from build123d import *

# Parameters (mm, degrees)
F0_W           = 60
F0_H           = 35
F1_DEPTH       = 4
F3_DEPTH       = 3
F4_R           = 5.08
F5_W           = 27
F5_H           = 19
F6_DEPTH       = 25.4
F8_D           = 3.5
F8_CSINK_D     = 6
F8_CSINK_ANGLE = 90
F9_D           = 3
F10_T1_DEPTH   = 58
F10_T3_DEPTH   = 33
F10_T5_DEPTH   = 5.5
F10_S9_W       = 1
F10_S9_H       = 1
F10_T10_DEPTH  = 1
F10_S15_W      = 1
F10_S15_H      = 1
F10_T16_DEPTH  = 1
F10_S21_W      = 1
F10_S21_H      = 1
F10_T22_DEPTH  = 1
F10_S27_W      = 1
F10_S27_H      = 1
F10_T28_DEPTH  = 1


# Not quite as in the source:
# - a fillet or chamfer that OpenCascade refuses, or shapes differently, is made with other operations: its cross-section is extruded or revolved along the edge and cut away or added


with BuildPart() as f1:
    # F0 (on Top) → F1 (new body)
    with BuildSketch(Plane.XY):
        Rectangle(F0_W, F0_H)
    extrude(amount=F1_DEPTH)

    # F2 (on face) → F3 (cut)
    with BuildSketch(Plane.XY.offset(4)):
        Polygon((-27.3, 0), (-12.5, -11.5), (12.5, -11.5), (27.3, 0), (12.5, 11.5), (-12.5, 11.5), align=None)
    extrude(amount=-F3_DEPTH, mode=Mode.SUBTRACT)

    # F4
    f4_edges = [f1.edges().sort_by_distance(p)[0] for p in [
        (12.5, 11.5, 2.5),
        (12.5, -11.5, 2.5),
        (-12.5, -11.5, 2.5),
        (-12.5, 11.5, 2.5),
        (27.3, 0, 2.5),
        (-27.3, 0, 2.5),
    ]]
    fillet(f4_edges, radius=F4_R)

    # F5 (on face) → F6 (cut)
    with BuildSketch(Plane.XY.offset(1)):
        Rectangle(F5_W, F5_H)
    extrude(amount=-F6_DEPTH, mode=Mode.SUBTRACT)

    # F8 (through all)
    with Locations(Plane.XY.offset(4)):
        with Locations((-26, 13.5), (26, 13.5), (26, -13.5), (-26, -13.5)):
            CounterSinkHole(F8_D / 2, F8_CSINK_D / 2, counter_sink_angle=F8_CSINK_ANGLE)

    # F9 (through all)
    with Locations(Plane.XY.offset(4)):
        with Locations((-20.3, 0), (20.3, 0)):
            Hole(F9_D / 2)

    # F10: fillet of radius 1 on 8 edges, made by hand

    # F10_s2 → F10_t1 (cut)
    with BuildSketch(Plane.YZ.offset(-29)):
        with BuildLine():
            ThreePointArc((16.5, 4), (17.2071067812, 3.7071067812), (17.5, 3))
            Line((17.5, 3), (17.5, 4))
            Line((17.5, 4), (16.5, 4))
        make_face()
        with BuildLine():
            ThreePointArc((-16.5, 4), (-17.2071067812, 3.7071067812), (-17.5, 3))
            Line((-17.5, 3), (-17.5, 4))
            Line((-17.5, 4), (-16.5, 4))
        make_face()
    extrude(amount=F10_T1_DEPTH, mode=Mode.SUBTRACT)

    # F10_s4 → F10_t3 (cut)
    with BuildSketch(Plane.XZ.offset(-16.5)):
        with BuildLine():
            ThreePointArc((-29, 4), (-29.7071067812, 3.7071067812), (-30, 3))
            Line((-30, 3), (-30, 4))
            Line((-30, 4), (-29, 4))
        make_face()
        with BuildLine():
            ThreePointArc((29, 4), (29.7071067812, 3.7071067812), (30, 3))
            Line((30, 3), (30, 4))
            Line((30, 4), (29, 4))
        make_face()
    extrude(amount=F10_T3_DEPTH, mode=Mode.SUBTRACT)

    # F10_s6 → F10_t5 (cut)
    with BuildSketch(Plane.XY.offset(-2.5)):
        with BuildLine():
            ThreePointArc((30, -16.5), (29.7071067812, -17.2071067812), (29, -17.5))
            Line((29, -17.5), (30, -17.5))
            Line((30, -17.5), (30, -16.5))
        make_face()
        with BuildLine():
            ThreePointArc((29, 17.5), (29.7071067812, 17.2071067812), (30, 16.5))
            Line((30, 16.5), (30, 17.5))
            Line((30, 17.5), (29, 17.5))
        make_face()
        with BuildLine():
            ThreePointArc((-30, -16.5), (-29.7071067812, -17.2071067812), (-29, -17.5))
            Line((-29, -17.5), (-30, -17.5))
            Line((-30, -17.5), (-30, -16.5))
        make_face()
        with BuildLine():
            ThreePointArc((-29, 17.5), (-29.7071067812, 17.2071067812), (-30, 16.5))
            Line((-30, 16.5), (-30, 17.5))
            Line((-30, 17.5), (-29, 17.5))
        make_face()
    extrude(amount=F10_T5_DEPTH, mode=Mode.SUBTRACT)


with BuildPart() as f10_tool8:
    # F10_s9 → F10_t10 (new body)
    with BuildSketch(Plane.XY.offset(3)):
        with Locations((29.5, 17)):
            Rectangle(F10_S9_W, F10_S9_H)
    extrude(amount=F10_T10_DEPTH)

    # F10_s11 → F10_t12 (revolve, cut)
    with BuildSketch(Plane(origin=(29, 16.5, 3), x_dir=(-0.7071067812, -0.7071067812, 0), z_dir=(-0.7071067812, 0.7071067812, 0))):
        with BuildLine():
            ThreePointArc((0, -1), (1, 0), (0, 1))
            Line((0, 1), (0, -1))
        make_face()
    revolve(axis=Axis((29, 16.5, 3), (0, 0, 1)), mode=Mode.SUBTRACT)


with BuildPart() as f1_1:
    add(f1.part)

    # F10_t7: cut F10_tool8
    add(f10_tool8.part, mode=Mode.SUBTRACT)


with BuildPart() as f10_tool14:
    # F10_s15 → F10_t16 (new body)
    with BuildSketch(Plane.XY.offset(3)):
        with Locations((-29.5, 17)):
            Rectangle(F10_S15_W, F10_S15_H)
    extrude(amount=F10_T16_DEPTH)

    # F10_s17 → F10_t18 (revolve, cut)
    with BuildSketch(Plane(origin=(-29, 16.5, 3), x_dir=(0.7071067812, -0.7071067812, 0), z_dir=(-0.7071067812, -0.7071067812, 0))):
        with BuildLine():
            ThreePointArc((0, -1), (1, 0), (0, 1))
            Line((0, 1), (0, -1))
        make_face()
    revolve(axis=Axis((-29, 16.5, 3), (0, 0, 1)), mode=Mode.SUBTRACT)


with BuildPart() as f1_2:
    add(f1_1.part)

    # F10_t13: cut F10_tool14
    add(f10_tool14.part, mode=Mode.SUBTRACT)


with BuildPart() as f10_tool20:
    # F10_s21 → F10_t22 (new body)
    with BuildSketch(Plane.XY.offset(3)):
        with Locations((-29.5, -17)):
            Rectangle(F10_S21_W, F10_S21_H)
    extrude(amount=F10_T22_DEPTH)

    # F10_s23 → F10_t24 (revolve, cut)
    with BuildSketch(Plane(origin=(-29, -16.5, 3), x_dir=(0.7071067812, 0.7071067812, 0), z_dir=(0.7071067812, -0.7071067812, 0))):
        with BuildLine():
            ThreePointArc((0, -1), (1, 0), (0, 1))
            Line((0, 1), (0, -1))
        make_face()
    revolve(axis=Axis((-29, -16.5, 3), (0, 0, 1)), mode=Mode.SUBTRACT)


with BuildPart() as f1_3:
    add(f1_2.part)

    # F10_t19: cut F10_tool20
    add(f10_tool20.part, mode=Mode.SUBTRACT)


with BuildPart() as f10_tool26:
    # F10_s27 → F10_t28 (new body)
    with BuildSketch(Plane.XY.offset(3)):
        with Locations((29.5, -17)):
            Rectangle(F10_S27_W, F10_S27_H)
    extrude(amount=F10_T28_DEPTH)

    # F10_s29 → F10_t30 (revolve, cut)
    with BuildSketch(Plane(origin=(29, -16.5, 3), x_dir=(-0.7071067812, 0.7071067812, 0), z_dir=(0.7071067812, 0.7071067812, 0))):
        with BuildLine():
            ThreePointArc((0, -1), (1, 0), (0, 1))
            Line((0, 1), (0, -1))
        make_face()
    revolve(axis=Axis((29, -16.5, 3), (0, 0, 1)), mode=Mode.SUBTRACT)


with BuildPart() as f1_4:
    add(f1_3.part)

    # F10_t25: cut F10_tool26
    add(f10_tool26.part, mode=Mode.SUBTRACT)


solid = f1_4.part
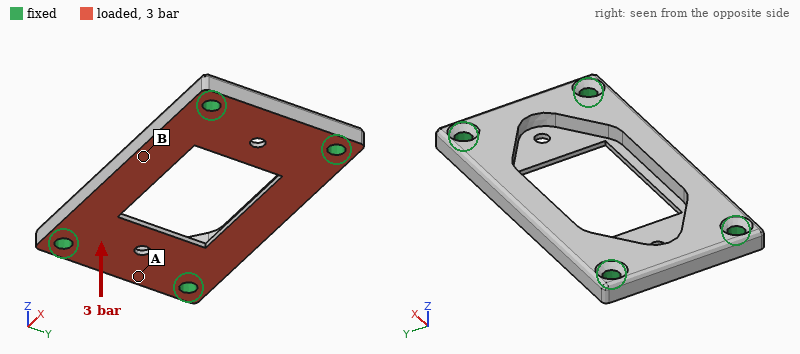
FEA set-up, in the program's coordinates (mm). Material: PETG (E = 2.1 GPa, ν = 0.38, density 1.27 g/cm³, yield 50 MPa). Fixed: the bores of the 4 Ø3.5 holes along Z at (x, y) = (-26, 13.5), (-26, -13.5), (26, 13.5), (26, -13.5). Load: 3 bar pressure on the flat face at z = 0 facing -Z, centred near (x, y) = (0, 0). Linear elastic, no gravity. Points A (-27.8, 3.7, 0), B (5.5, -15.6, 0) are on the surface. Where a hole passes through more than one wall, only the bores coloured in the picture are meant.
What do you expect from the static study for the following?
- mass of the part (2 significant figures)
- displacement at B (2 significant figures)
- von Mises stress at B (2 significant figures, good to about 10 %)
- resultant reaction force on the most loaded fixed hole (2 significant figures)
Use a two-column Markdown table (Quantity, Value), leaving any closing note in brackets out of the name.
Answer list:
| Quantity | Value |
|---|---|
| mass of the part | 6.3 g |
| displacement at B | 0.55 mm |
| von Mises stress at B | 12 MPa |
| resultant reaction force on the most loaded fixed hole | 120 N |
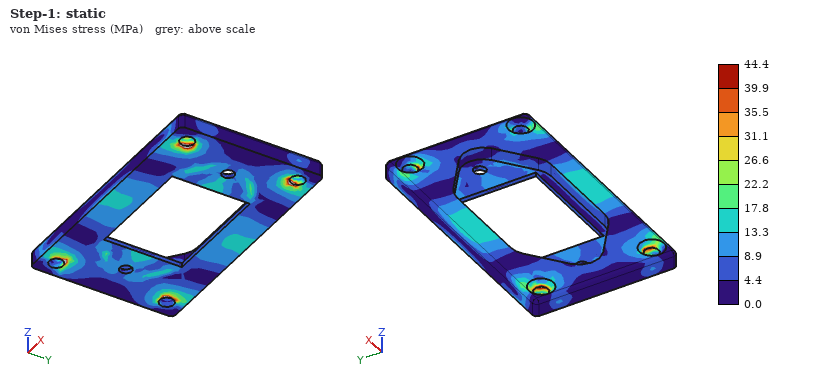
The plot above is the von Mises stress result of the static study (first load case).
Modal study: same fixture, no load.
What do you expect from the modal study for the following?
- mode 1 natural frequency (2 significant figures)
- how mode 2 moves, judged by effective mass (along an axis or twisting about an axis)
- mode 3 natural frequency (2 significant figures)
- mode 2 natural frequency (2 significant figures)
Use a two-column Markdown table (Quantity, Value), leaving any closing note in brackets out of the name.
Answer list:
| Quantity | Value |
|---|---|
| mode 1 natural frequency | 2100 Hz |
| how mode 2 moves, judged by effective mass | twisting about X |
| mode 3 natural frequency | 4200 Hz |
| mode 2 natural frequency | 2100 Hz |
